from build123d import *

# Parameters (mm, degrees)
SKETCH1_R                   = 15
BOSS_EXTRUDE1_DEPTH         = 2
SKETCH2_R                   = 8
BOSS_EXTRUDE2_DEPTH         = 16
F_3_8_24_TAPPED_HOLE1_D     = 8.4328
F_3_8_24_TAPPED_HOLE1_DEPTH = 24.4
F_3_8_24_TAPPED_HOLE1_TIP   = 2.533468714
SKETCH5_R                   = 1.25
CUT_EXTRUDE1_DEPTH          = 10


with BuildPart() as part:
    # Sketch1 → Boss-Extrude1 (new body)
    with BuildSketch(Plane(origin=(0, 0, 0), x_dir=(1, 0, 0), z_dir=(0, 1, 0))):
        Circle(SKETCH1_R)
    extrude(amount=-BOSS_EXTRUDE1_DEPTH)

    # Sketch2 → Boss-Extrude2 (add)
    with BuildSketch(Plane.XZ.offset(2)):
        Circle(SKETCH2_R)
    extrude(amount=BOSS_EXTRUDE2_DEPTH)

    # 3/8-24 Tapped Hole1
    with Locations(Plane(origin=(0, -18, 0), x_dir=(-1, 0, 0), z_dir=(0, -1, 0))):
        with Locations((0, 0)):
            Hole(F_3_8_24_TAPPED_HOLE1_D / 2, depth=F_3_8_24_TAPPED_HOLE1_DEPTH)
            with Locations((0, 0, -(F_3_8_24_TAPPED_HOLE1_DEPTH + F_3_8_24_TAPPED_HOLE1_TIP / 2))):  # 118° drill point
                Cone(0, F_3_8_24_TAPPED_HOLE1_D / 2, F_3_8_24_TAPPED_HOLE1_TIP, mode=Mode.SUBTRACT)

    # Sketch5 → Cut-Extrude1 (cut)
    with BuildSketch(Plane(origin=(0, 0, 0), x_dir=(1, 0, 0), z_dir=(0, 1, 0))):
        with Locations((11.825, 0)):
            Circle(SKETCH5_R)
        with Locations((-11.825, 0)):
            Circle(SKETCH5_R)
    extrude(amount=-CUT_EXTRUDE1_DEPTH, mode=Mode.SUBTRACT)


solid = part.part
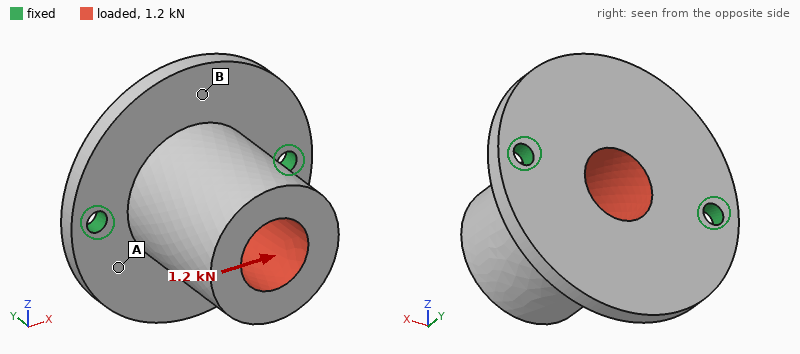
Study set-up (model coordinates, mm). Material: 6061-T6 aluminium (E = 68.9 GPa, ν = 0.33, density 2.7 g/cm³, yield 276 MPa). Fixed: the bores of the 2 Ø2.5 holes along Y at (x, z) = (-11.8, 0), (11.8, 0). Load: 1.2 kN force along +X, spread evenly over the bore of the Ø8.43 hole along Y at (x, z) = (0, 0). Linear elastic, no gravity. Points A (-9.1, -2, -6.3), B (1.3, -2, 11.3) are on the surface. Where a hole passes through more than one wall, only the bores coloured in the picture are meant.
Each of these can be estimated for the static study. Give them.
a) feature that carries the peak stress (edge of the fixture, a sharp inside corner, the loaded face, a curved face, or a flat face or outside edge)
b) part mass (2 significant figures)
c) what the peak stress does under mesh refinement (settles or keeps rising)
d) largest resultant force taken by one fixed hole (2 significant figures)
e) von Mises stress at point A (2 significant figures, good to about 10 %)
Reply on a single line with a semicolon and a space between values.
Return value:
edge of the fixture; 9.7 g; keeps rising; 780 N; 33 MPa
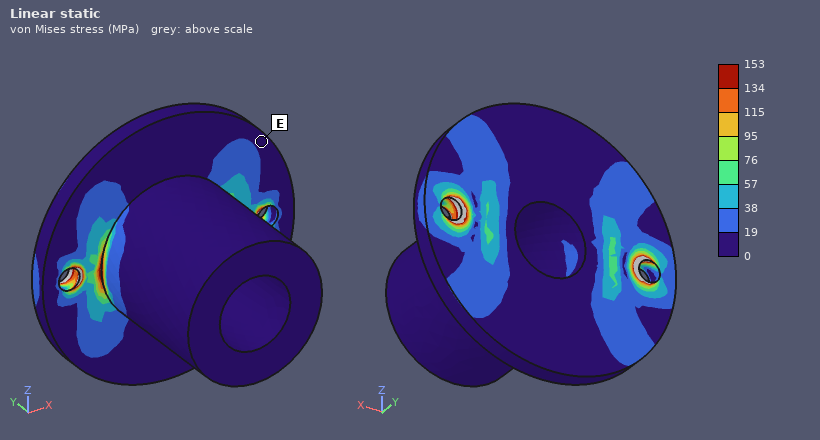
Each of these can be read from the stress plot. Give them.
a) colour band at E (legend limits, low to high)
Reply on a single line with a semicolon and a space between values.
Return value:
0 to 19 MPa
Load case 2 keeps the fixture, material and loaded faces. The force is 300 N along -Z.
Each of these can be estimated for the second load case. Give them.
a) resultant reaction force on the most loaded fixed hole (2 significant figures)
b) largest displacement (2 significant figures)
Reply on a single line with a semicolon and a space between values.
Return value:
150 N; 95 µm
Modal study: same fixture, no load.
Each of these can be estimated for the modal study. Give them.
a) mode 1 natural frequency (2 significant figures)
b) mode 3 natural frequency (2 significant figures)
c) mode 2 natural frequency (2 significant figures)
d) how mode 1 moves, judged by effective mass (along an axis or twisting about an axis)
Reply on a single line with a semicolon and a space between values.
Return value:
3600 Hz; 12 kHz; 12 kHz; along Z
